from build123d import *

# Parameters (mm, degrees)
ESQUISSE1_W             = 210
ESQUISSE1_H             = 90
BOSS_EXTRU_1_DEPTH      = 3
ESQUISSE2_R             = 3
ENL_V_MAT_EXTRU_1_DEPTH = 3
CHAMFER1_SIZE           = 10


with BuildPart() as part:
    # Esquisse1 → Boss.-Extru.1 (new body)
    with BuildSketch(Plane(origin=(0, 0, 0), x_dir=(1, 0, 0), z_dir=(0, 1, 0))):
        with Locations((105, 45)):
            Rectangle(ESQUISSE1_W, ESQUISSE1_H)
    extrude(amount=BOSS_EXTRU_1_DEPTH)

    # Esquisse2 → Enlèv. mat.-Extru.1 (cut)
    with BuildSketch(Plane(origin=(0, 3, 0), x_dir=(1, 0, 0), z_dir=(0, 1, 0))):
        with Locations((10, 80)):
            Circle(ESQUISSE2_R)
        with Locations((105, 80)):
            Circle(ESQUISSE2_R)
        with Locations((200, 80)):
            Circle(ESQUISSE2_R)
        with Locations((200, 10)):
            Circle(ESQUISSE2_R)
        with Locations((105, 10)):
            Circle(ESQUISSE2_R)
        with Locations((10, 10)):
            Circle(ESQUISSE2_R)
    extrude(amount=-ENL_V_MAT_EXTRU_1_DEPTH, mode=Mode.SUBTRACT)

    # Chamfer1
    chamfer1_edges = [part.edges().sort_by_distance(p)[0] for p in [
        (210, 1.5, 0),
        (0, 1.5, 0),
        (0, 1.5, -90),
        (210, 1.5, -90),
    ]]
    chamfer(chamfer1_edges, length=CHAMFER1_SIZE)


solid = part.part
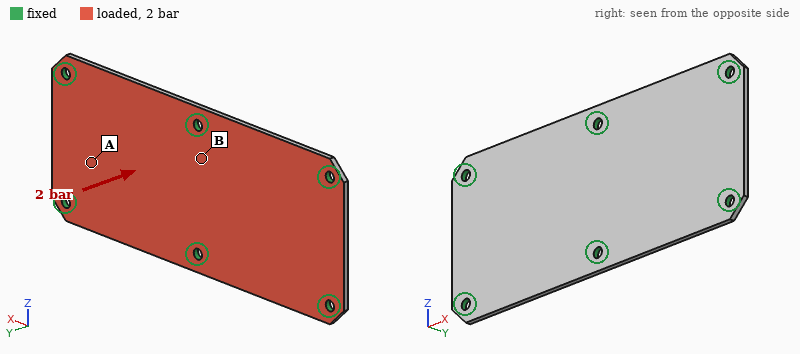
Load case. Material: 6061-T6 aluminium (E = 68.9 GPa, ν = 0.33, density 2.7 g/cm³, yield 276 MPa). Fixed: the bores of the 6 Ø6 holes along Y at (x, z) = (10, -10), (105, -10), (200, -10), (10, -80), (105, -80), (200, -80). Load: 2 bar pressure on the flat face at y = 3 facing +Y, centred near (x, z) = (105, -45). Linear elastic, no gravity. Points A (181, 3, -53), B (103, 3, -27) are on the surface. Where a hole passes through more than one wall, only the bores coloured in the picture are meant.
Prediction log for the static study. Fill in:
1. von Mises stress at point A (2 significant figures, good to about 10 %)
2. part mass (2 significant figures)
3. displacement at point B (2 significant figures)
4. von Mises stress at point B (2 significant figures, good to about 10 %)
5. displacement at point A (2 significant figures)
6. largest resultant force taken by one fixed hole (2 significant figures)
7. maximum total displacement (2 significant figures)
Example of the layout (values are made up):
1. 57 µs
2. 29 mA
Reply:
1. 28 MPa
2. 150 g
3. 0.092 mm
4. 66 MPa
5. 0.22 mm
6. 880 N
7. 0.36 mm
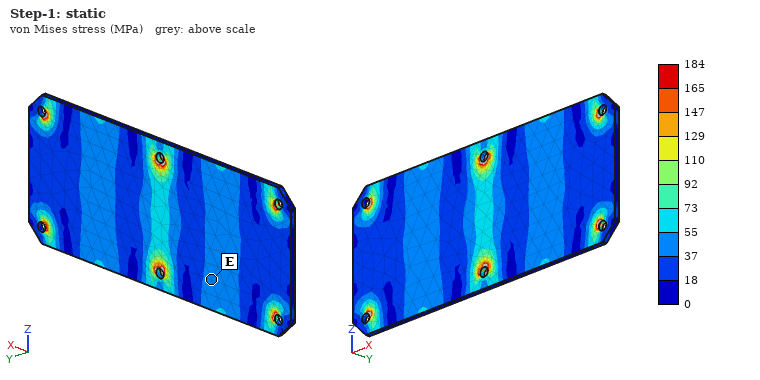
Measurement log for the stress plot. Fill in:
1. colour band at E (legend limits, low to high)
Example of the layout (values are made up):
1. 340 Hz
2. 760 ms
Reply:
1. 37 to 55 MPa
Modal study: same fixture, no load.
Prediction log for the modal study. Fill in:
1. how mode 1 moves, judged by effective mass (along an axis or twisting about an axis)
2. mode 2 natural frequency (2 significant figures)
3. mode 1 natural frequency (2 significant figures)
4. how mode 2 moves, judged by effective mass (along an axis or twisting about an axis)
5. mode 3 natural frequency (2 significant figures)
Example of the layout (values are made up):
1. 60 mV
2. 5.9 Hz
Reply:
1. twisting about Z
2. 1600 Hz
3. 1500 Hz
4. along Y
5. 2200 Hz
